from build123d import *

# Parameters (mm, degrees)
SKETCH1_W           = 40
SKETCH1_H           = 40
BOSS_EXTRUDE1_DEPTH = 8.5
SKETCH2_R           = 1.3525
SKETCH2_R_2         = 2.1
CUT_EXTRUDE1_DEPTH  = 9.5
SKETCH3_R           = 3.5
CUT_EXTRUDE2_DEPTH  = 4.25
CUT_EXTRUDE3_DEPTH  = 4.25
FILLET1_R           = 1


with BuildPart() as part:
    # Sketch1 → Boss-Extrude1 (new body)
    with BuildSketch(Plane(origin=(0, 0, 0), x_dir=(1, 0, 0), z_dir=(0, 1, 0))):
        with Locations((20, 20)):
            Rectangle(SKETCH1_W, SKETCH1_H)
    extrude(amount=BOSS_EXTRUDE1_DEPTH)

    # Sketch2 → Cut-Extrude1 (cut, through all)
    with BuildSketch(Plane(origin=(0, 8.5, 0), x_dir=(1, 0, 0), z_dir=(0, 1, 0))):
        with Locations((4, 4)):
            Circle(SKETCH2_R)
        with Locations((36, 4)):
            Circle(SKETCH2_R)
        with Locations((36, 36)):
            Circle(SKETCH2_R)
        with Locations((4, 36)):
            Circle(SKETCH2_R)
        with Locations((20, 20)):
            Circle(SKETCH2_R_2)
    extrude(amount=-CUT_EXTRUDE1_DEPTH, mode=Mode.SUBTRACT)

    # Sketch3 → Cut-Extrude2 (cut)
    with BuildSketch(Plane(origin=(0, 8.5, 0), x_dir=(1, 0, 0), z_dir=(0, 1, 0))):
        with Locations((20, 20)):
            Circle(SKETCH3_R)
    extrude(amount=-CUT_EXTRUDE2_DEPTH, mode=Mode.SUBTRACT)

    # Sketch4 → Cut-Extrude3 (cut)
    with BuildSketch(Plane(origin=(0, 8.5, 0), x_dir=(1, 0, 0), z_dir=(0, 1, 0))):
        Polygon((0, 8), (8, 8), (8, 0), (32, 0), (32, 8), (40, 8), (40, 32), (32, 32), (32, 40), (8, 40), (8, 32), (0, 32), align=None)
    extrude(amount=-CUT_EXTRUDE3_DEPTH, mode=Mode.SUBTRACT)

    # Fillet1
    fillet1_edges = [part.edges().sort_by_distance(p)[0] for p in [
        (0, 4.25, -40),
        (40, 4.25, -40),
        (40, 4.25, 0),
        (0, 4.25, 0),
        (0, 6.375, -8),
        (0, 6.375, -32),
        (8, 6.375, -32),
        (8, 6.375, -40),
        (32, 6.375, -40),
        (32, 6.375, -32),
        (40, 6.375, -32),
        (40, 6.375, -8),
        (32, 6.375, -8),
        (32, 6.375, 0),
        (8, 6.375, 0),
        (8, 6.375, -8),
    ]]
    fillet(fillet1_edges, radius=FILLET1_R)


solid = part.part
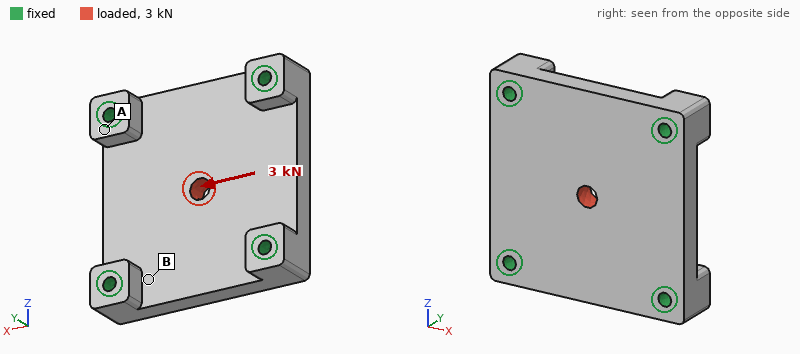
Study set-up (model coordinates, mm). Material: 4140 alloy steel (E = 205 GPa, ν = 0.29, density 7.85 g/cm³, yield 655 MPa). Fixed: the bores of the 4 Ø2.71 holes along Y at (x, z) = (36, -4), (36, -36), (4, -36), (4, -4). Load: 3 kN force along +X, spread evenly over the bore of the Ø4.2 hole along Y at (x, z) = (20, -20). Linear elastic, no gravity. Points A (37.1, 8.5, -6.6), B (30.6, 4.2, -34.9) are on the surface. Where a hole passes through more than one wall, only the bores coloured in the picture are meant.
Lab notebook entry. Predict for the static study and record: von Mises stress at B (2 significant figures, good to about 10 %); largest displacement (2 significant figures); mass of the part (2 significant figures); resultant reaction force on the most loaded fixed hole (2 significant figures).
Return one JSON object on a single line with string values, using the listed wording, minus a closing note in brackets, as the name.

{"von Mises stress at B": "21 MPa", "largest displacement": "3.1 µm", "mass of the part": "60 g", "resultant reaction force on the most loaded fixed hole": "840 N"}
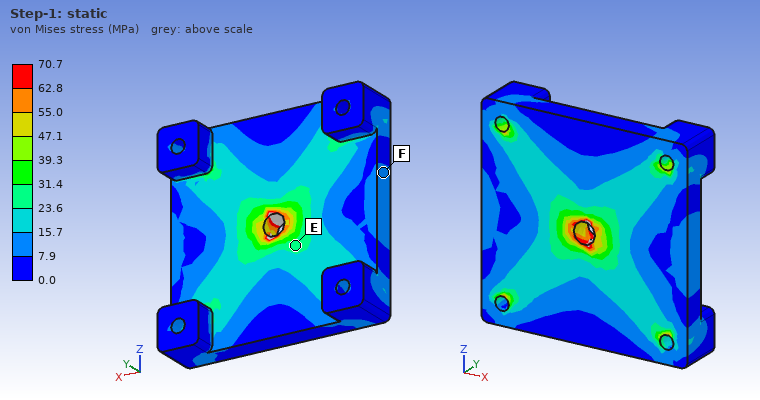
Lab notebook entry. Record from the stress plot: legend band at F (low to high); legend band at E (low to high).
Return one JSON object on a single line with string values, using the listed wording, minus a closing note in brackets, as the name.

{"legend band at F": "7.9 to 15.7 MPa", "legend band at E": "23.6 to 31.4 MPa"}
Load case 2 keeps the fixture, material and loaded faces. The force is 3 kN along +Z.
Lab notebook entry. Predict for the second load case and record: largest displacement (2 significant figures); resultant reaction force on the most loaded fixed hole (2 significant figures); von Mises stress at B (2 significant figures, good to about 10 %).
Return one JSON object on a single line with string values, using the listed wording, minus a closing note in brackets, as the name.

{"largest displacement": "3.1 µm", "resultant reaction force on the most loaded fixed hole": "840 N", "von Mises stress at B": "21 MPa"}
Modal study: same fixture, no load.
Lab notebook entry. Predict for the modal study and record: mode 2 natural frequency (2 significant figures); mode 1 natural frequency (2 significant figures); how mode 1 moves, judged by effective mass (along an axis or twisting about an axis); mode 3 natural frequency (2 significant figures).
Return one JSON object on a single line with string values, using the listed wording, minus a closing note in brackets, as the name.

{"mode 2 natural frequency": "26 kHz", "mode 1 natural frequency": "16 kHz", "how mode 1 moves, judged by effective mass": "along Y", "mode 3 natural frequency": "26 kHz"}
